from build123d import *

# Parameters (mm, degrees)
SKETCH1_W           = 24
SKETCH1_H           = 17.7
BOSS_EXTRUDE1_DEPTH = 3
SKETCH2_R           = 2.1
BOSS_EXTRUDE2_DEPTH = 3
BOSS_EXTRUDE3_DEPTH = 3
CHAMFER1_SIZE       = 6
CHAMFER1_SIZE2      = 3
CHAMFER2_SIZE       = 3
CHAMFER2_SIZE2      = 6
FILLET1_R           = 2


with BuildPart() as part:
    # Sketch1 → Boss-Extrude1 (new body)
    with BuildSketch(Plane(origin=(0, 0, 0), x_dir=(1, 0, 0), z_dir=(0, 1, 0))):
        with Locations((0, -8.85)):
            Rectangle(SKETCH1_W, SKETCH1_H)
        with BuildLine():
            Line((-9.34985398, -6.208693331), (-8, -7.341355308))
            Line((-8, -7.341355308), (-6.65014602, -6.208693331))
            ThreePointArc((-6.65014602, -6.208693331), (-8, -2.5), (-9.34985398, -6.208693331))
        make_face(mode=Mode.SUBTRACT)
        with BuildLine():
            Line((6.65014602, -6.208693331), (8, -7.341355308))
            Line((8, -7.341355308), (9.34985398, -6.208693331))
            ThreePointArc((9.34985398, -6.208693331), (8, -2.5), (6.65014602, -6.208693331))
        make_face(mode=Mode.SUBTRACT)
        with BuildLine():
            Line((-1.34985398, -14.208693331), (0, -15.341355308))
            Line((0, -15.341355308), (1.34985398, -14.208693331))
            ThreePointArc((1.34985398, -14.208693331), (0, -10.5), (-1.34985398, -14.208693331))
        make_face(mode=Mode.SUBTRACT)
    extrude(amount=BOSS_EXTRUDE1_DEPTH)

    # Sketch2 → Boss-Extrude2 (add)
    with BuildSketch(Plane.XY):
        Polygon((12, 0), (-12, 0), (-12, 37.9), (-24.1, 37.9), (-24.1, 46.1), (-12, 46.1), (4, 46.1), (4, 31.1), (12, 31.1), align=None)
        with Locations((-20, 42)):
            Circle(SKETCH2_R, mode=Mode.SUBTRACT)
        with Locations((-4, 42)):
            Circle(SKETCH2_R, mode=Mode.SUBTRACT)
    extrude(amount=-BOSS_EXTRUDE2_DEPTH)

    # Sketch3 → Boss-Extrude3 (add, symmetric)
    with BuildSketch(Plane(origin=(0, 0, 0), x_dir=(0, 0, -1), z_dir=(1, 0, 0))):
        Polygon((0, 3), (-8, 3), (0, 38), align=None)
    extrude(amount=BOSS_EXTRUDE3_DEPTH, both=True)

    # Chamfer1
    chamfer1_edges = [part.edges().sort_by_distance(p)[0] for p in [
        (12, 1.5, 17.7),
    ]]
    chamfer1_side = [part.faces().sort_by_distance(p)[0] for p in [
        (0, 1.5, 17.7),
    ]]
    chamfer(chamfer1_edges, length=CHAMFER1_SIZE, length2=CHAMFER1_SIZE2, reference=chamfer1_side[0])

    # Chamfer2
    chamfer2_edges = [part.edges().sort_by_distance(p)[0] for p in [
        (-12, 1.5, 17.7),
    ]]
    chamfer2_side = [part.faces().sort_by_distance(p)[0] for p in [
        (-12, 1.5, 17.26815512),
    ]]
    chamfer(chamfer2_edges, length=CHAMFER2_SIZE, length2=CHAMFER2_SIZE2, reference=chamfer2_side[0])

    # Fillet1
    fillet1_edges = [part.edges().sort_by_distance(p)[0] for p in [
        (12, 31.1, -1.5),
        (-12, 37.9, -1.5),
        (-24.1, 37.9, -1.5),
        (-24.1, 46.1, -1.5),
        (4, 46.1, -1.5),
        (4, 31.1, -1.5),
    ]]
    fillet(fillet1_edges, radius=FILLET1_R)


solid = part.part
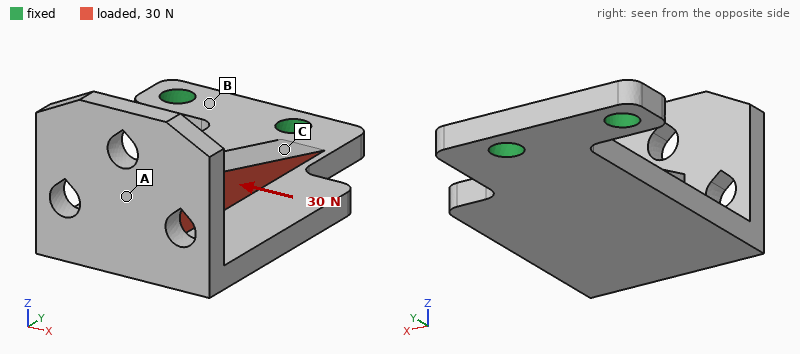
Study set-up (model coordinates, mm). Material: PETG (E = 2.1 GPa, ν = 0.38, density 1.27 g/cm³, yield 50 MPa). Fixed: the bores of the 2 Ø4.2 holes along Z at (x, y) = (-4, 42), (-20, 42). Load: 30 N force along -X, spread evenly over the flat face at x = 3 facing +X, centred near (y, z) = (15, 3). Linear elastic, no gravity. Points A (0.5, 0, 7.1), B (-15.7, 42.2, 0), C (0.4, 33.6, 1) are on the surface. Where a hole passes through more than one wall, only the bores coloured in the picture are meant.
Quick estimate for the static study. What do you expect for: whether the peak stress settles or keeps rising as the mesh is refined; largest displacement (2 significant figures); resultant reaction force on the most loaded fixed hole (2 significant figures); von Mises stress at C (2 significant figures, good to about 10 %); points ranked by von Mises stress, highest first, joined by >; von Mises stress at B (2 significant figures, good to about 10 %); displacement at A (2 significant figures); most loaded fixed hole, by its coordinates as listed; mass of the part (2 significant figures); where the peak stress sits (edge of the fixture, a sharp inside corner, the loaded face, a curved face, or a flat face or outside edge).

keeps rising
0.59 mm
41 N
3.6 MPa
C > B > A
2.4 MPa
0.40 mm
(-20, 42)
6.5 g
edge of the fixture
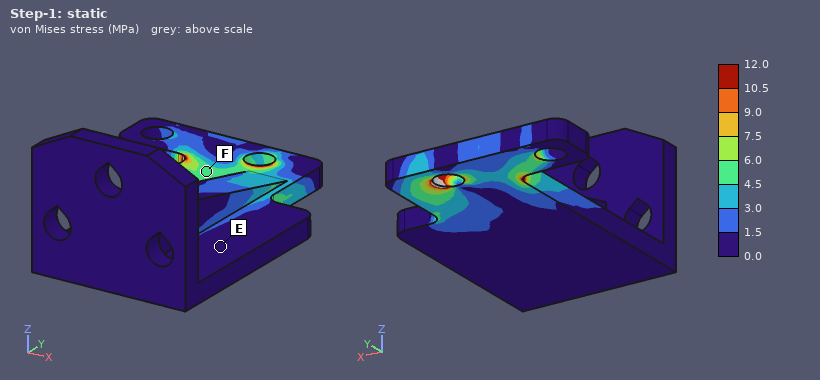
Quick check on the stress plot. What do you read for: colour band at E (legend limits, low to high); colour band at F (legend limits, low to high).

0.0 to 1.5 MPa
4.5 to 6.0 MPa
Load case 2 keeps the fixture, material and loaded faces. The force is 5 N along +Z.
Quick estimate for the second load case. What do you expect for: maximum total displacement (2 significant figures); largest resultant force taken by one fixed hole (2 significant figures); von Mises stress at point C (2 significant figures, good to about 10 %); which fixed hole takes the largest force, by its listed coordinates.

0.64 mm
7.1 N
3.0 MPa
(-4, 42)
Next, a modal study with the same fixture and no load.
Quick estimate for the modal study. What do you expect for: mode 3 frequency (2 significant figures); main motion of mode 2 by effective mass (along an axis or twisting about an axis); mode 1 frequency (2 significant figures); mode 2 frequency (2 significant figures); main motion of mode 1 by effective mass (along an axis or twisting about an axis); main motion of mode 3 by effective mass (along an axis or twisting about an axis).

990 Hz
along X
220 Hz
610 Hz
along Z
along X
